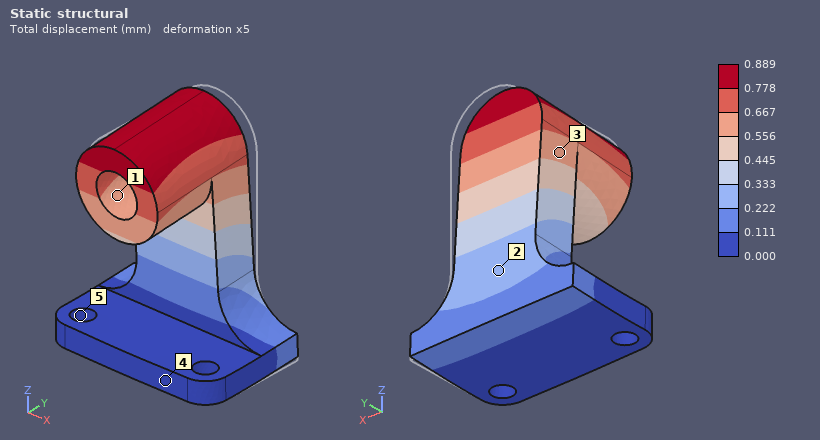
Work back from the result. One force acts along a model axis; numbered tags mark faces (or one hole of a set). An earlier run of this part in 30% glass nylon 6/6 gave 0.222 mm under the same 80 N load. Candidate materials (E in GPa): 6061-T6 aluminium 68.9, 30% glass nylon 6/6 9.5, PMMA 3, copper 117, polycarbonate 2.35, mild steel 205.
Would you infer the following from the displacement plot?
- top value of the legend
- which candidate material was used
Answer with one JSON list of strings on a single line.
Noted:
["0.889 mm", "polycarbonate"]
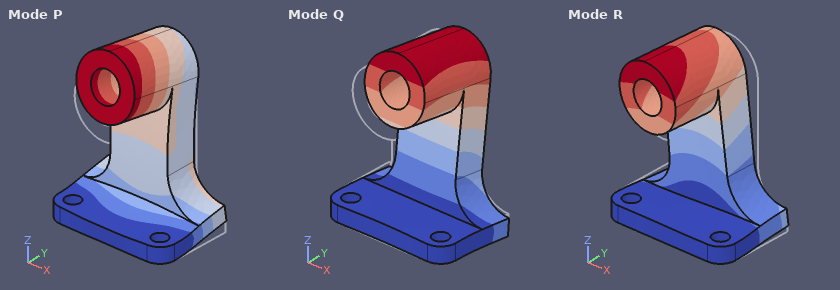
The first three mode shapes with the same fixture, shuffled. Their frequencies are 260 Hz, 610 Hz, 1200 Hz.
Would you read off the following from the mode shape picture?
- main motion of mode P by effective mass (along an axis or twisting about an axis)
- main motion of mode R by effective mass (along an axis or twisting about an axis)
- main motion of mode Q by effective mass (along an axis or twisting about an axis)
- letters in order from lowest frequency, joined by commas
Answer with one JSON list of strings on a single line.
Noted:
["along Z", "along X", "along Y", "Q, R, P"]
